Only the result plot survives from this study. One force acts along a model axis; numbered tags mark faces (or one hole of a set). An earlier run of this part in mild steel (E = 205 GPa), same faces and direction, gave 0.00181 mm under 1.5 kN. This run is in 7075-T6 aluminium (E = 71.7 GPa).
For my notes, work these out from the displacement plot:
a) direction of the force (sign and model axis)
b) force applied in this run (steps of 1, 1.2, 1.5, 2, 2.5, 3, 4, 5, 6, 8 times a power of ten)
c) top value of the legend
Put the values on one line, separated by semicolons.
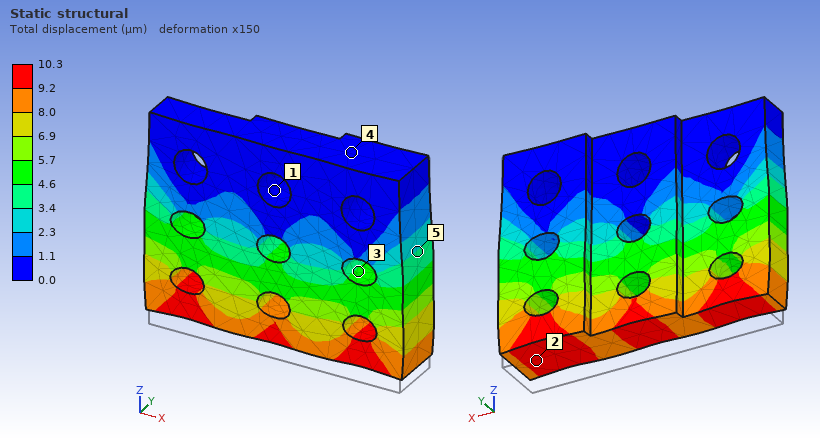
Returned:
+Z; 3 kN; 10.3 µm
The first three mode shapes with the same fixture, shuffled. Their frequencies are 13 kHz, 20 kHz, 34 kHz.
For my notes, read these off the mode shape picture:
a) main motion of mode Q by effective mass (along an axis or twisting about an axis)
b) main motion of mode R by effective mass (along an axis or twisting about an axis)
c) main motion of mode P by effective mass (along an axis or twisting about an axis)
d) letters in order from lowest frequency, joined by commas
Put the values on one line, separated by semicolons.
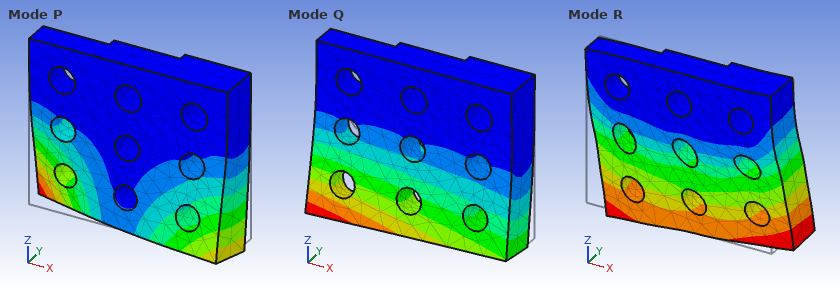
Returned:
along Y; along X; twisting about Z; Q, P, R
